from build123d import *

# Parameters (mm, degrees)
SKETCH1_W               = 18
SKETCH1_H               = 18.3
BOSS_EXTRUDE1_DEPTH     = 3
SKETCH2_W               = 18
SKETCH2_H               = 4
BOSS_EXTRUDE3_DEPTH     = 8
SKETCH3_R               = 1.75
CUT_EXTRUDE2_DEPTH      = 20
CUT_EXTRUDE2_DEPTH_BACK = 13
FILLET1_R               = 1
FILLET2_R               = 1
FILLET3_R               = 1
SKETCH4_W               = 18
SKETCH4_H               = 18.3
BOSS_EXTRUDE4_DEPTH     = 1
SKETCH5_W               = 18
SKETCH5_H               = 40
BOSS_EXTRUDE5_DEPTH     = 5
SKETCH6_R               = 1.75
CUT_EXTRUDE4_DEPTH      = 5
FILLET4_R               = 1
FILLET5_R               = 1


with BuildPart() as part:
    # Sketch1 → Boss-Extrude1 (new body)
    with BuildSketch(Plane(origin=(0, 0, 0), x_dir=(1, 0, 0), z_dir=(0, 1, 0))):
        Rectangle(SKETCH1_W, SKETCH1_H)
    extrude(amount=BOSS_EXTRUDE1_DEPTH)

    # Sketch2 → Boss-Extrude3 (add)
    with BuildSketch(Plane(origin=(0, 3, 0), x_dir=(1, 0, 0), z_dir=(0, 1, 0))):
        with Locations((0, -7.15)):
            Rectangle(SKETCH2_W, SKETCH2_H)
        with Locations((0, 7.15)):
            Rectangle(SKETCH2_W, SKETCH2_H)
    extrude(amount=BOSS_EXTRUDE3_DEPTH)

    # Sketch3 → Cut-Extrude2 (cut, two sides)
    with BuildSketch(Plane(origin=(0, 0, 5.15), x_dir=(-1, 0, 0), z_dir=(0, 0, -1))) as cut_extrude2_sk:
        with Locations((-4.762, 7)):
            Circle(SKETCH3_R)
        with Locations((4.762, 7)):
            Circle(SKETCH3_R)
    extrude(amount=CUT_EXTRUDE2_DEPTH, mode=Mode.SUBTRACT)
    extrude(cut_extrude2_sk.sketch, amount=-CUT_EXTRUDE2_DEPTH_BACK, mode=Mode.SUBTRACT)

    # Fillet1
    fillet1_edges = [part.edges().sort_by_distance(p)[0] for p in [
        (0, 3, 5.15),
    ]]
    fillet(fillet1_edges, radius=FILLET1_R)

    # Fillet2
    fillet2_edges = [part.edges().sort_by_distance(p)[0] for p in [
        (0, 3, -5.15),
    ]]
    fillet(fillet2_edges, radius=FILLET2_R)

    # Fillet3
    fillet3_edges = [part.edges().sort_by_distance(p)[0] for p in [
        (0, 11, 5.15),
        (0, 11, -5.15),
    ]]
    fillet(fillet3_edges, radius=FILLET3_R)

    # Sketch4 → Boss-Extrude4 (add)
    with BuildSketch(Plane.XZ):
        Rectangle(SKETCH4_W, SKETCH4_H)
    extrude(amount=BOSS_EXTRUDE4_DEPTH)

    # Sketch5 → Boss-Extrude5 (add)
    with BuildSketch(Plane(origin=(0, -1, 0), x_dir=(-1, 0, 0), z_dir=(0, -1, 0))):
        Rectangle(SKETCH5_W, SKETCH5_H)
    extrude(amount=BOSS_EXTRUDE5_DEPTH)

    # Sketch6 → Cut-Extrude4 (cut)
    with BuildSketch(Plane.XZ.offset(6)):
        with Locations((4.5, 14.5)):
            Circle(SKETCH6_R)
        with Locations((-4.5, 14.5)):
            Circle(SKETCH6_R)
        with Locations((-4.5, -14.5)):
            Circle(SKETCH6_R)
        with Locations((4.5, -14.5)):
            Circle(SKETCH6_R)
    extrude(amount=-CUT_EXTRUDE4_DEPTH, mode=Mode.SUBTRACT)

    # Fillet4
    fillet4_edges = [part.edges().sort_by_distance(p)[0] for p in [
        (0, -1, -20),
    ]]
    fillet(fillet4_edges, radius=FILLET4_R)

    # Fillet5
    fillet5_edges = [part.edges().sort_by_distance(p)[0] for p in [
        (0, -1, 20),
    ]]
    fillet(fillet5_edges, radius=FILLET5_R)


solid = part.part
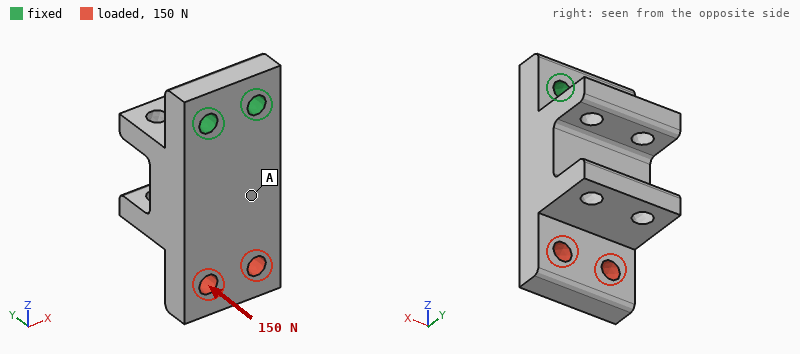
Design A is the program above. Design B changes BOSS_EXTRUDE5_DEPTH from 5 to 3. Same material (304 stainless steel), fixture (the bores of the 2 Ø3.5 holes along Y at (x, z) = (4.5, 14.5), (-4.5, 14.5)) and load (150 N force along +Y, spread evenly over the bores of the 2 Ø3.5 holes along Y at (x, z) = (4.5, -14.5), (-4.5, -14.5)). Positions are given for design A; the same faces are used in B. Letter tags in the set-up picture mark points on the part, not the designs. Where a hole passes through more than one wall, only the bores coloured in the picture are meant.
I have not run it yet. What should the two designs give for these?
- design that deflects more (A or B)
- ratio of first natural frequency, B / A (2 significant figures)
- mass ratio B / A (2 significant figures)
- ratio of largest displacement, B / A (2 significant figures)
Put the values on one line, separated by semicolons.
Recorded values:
B; 0.61; 0.76; 3.7
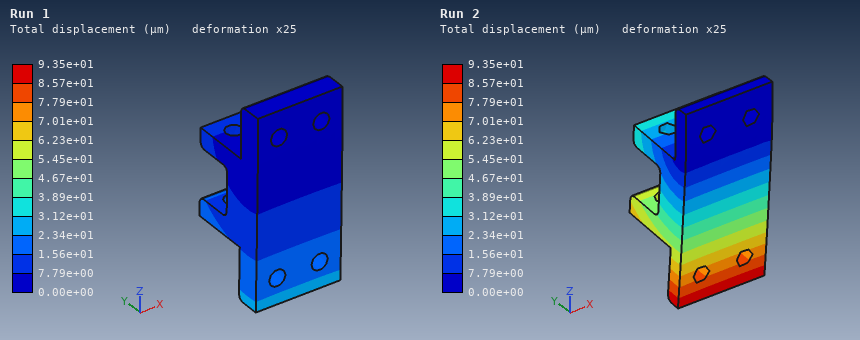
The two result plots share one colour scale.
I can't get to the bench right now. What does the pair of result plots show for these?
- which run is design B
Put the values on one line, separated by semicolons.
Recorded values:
Run 2
